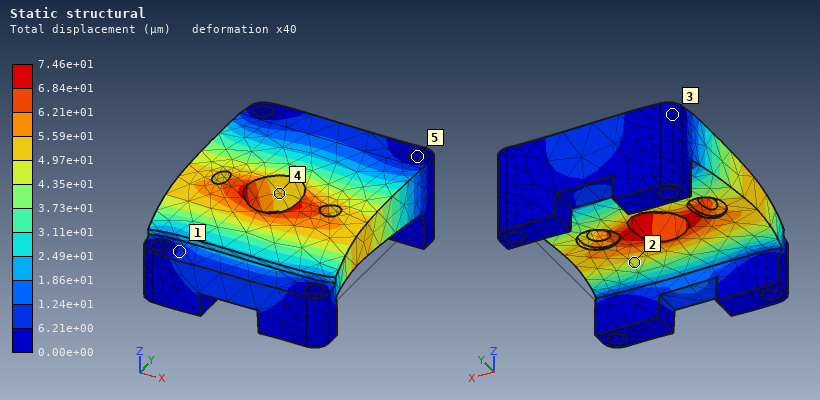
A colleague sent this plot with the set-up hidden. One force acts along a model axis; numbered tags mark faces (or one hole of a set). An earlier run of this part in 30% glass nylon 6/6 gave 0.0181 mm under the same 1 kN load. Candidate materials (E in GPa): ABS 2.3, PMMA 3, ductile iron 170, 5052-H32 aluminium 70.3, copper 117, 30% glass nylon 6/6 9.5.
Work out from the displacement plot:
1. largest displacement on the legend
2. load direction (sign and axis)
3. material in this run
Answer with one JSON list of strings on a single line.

["7.46e+01 µm", "-X", "ABS"]
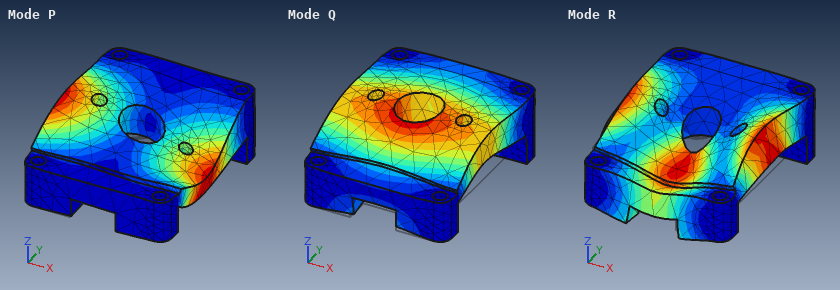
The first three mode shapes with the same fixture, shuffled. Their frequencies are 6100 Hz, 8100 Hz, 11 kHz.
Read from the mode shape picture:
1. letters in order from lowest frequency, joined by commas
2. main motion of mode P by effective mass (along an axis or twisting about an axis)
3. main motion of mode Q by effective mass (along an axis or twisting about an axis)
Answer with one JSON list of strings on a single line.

["Q, P, R", "twisting about Y", "along Z"]
